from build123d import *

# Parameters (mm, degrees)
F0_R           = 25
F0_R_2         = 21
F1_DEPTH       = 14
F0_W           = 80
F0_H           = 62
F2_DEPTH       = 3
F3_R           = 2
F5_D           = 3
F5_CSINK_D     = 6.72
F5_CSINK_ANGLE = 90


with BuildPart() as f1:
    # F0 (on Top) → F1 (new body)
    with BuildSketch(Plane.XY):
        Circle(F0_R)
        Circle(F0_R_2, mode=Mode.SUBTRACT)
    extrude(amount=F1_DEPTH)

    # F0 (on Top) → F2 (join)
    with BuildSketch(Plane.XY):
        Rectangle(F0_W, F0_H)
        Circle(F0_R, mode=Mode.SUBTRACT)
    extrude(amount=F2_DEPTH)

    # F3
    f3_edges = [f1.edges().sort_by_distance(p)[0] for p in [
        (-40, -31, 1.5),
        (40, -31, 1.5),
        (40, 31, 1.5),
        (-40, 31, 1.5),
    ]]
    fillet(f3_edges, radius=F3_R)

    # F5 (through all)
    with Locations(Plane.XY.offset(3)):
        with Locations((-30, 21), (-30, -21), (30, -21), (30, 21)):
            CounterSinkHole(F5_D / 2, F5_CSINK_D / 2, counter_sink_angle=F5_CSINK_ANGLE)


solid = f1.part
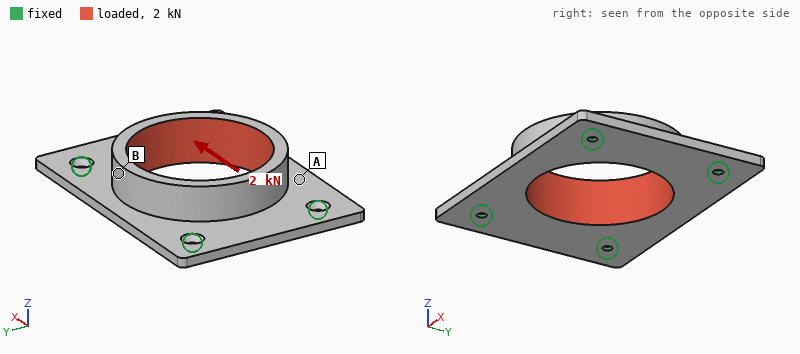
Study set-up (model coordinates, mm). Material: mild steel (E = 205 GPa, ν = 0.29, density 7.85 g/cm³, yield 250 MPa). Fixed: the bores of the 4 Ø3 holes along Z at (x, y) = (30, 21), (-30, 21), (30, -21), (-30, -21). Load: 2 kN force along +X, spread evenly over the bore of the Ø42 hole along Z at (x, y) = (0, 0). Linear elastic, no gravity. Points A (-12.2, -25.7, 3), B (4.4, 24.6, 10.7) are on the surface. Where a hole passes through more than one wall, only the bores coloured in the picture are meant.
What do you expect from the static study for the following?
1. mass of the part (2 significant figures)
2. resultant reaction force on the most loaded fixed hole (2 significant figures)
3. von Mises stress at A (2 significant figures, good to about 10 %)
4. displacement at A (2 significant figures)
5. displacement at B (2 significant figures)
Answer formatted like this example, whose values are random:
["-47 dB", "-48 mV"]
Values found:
["130 g", "520 N", "11 MPa", "1.3 µm", "2.2 µm"]
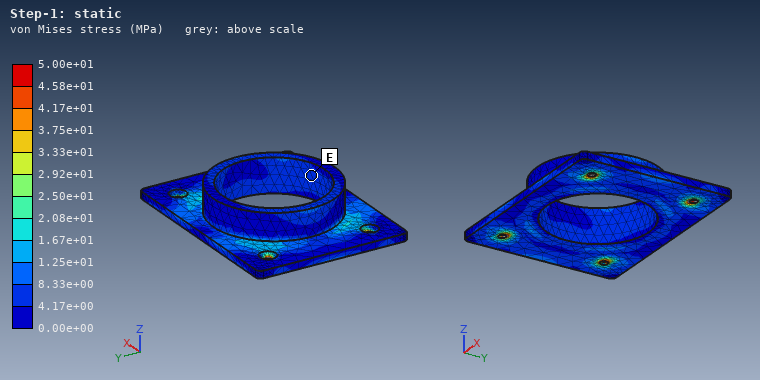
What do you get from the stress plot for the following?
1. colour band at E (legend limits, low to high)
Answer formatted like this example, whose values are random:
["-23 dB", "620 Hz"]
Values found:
["4.17e+00 to 8.33e+00 MPa"]
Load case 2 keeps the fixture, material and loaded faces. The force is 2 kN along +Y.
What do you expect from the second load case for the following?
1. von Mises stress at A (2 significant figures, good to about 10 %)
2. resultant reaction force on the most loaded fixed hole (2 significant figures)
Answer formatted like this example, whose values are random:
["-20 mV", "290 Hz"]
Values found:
["15 MPa", "560 N"]
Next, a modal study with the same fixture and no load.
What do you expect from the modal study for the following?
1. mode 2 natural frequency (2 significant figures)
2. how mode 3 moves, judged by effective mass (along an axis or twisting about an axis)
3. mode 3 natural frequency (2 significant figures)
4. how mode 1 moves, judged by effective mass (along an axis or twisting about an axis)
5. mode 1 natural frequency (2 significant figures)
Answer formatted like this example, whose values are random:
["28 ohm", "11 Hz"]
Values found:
["4800 Hz", "twisting about Y", "7100 Hz", "along Z", "4400 Hz"]
